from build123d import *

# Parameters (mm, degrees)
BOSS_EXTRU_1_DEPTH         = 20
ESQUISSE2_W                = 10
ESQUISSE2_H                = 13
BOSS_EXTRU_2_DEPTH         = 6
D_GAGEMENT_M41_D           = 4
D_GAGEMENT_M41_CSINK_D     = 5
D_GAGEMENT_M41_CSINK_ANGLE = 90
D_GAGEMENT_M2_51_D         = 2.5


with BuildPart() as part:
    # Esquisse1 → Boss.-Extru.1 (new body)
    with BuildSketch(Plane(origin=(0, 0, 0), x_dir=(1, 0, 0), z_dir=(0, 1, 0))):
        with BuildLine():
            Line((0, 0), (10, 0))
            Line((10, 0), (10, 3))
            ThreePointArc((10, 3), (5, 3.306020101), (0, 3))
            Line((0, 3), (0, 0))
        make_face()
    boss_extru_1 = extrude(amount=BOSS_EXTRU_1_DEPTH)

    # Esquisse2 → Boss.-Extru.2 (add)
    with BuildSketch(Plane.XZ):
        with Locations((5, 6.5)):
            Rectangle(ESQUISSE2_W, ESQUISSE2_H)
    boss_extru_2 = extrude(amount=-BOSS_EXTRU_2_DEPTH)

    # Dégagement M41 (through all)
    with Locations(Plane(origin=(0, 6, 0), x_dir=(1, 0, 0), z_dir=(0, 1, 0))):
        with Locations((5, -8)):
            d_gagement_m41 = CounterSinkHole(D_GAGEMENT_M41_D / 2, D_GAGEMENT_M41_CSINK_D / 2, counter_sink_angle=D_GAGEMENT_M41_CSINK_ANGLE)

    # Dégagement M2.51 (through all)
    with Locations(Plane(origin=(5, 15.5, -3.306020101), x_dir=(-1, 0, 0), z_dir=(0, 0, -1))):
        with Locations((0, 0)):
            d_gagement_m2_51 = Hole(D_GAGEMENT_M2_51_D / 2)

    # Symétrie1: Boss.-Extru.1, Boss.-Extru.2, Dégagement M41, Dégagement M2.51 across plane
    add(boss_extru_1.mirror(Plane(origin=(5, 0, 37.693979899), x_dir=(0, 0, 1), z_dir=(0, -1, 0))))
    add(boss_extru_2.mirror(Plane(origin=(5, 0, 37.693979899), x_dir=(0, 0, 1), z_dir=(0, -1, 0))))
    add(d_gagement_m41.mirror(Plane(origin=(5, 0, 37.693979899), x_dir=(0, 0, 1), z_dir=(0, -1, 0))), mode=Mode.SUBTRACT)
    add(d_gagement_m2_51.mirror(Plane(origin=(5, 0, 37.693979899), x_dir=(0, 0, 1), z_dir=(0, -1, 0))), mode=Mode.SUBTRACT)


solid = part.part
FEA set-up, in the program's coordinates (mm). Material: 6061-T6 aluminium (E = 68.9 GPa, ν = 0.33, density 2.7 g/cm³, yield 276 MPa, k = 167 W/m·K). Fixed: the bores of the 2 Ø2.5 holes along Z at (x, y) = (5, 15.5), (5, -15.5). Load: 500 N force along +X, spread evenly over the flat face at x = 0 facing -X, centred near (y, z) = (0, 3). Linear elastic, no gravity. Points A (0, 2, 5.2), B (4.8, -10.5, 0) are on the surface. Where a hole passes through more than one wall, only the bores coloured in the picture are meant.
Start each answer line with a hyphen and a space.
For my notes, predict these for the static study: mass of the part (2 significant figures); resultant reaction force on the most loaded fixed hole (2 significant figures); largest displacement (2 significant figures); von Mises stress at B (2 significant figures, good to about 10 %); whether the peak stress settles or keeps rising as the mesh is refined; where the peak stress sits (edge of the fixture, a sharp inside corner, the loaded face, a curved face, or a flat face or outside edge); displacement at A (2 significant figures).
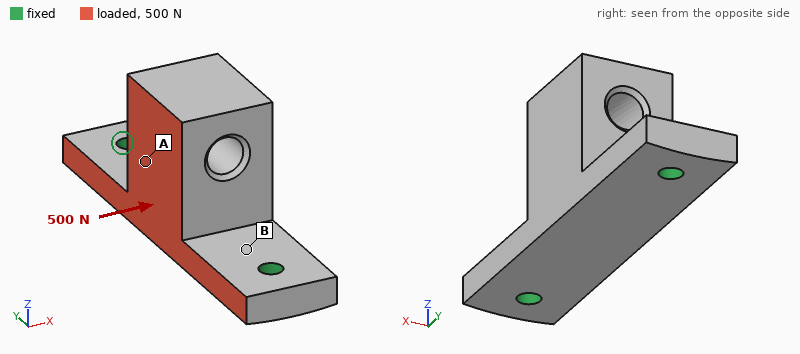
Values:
- 7.2 g
- 250 N
- 79 µm
- 75 MPa
- keeps rising
- edge of the fixture
- 46 µm
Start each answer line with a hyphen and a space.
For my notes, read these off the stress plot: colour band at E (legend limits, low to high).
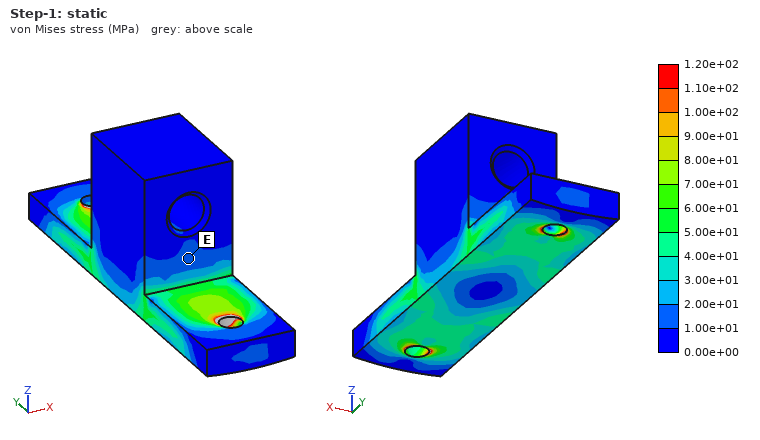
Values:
- 1.00e+01 to 2.00e+01 MPa
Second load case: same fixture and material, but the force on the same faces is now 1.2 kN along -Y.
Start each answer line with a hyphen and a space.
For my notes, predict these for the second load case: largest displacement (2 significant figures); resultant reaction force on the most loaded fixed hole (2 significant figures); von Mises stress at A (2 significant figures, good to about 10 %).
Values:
- 36 µm
- 680 N
- 26 MPa
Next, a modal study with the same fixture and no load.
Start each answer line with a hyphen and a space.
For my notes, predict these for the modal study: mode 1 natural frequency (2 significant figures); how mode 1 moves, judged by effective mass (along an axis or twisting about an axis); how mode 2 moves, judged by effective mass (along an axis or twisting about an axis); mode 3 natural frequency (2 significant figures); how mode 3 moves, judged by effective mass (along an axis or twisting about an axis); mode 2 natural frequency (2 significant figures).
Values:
- 5800 Hz
- along X
- along Z
- 14 kHz
- along Y
- 11 kHz
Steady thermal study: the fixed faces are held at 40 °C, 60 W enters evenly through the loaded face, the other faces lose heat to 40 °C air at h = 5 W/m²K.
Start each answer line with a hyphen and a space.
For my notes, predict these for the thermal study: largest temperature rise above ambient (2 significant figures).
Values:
- 69 K
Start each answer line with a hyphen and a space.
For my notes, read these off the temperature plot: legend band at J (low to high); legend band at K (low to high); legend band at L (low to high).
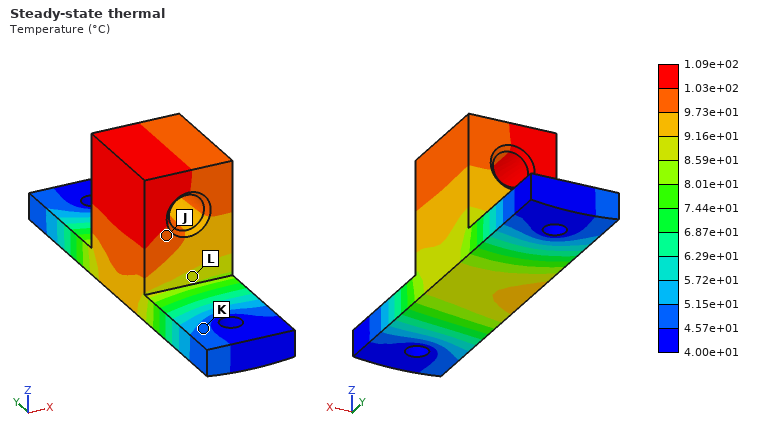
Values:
- 9.73e+01 to 1.03e+02 °C
- 4.57e+01 to 5.15e+01 °C
- 8.59e+01 to 9.16e+01 °C
